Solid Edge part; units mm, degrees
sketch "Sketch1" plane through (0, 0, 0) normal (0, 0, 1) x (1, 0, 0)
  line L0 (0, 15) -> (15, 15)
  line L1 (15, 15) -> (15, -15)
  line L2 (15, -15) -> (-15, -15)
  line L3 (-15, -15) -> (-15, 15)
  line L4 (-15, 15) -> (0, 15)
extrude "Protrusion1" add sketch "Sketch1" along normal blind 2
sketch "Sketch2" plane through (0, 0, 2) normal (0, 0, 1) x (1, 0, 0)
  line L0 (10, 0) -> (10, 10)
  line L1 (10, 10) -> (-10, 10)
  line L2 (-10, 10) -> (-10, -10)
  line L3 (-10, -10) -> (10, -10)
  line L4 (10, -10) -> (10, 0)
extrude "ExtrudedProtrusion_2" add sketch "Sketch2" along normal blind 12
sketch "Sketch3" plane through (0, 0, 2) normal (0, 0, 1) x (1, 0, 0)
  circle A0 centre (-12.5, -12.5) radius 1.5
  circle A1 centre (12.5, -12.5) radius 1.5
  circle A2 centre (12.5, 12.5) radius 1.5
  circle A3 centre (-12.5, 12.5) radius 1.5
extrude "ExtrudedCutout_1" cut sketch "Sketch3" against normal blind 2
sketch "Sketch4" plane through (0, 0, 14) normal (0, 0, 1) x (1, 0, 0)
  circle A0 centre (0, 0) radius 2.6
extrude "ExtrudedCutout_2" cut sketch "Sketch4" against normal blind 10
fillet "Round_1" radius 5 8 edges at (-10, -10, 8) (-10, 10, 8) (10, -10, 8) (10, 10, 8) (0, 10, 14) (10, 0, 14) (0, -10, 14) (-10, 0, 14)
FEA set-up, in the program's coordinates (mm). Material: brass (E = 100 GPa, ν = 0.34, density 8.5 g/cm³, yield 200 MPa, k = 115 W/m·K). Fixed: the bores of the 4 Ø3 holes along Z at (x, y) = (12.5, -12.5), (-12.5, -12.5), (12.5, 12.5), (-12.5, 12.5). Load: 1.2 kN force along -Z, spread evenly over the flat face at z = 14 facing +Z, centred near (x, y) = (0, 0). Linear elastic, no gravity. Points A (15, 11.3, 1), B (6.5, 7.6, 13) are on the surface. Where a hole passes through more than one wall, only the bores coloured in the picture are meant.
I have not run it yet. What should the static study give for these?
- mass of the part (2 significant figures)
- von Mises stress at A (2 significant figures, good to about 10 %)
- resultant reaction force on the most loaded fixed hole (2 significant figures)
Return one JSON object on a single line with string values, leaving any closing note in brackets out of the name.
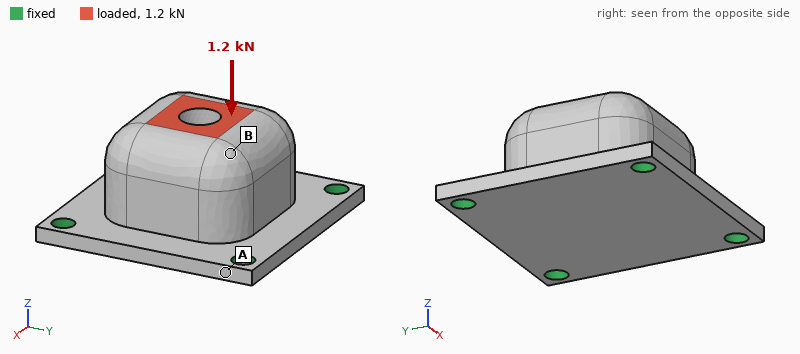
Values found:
{"mass of the part": "49 g", "von Mises stress at A": "35 MPa", "resultant reaction force on the most loaded fixed hole": "330 N"}
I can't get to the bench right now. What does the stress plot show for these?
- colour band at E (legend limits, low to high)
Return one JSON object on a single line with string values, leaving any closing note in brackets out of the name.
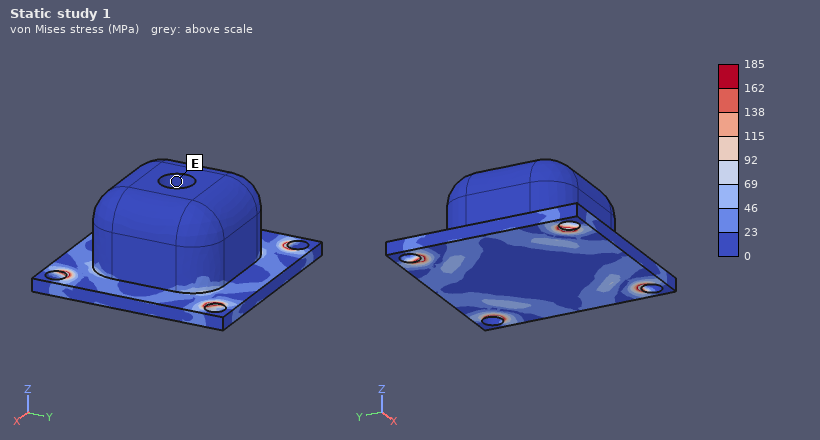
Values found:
{"colour band at E": "0 to 23 MPa"}
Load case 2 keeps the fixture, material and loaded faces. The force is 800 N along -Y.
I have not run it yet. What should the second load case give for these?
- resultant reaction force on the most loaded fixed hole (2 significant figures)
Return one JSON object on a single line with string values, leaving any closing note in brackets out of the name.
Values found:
{"resultant reaction force on the most loaded fixed hole": "340 N"}
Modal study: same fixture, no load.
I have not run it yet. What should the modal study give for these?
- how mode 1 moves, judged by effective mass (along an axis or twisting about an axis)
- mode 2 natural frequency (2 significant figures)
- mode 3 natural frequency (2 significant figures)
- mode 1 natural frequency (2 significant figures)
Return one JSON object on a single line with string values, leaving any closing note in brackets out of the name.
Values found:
{"how mode 1 moves, judged by effective mass": "along Z", "mode 2 natural frequency": "8400 Hz", "mode 3 natural frequency": "8400 Hz", "mode 1 natural frequency": "7200 Hz"}
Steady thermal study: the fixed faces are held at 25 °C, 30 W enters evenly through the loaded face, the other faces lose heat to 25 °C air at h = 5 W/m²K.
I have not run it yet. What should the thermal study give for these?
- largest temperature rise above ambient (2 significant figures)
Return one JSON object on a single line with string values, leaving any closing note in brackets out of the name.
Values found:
{"largest temperature rise above ambient": "38 K"}
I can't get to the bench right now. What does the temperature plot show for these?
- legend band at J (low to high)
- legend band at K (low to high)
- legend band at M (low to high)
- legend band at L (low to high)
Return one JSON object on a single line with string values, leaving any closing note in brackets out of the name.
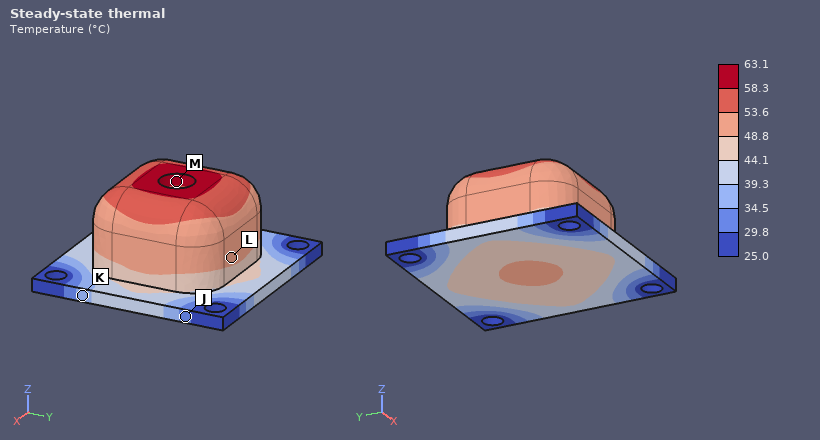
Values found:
{"legend band at J": "29.8 to 34.5 °C", "legend band at K": "34.5 to 39.3 °C", "legend band at M": "58.3 to 63.1 °C", "legend band at L": "48.8 to 53.6 °C"}
